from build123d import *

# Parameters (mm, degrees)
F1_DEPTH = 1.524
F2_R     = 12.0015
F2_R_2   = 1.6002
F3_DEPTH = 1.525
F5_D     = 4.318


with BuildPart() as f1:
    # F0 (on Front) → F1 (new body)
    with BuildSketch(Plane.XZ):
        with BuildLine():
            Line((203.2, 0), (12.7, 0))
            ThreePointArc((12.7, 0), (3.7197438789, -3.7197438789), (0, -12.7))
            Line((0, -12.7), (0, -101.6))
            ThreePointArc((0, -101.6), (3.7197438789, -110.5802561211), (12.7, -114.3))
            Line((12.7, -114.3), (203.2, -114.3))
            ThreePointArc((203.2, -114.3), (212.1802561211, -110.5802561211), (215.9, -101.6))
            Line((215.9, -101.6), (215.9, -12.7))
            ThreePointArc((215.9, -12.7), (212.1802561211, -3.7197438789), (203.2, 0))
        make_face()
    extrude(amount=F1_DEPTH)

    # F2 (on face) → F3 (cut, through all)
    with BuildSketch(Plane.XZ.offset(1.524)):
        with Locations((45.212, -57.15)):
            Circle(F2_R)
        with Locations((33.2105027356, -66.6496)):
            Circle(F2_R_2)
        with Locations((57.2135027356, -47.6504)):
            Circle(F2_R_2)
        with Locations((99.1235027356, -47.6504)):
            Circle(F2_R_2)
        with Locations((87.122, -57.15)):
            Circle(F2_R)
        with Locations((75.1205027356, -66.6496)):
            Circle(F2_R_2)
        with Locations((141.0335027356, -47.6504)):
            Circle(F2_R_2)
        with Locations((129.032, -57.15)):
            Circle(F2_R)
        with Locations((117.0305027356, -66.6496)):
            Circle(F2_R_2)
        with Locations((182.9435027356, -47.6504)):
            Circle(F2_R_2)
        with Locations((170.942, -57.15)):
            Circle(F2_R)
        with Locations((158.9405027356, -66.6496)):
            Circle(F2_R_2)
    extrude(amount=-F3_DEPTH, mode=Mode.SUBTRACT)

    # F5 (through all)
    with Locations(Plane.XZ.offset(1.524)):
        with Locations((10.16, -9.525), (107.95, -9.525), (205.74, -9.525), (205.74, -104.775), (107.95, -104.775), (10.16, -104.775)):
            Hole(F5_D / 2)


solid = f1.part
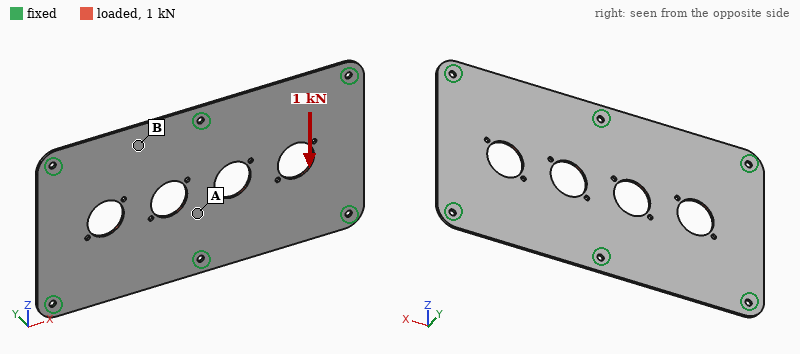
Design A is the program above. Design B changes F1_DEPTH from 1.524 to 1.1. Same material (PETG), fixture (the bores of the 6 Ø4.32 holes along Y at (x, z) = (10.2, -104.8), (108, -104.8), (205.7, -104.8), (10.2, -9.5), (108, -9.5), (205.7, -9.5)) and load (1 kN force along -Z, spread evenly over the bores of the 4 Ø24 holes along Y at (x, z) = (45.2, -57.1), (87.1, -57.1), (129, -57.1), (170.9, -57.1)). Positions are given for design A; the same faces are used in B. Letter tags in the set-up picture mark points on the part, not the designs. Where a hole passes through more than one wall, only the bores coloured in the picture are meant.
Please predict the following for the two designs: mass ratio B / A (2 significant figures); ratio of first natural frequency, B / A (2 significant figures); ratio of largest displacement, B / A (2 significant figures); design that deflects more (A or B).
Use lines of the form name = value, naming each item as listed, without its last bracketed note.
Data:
mass ratio B / A = 0.72
ratio of first natural frequency, B / A = 0.73
ratio of largest displacement, B / A = 1.4
design that deflects more = B
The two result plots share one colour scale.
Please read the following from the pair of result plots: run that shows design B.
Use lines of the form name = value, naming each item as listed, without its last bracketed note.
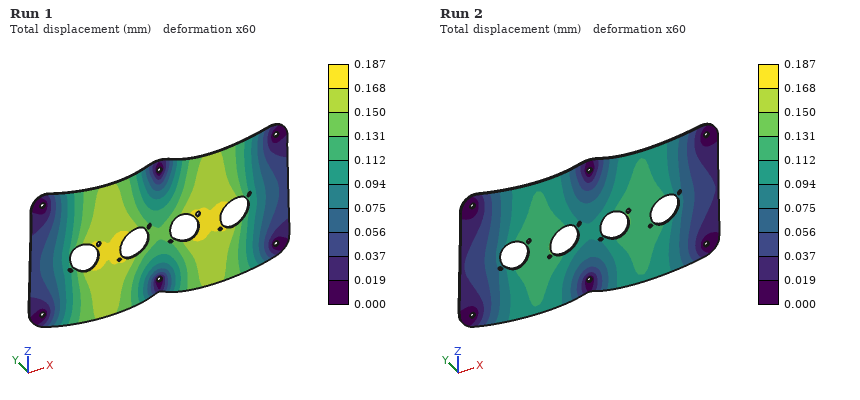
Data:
run that shows design B = Run 1
